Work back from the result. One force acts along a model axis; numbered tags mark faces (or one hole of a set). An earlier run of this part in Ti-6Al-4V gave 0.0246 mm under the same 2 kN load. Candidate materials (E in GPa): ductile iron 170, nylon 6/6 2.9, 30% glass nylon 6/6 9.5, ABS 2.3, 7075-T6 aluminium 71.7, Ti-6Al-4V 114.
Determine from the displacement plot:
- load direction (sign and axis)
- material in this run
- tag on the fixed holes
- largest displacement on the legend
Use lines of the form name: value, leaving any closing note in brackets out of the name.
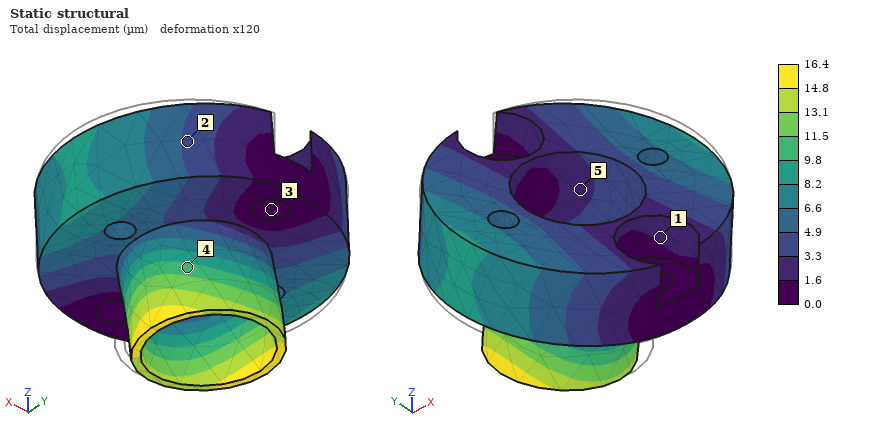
load direction: -X
material in this run: ductile iron
tag on the fixed holes: 3
largest displacement on the legend: 16.4 µm
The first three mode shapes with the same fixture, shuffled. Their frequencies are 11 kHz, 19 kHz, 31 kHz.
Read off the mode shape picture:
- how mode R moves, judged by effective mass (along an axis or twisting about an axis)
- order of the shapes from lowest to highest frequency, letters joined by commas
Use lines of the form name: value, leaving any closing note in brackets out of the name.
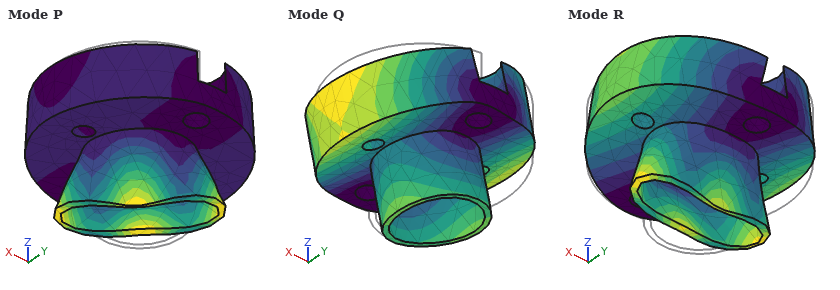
how mode R moves, judged by effective mass: along Z
order of the shapes from lowest to highest frequency, letters joined by commas: Q, R, P
